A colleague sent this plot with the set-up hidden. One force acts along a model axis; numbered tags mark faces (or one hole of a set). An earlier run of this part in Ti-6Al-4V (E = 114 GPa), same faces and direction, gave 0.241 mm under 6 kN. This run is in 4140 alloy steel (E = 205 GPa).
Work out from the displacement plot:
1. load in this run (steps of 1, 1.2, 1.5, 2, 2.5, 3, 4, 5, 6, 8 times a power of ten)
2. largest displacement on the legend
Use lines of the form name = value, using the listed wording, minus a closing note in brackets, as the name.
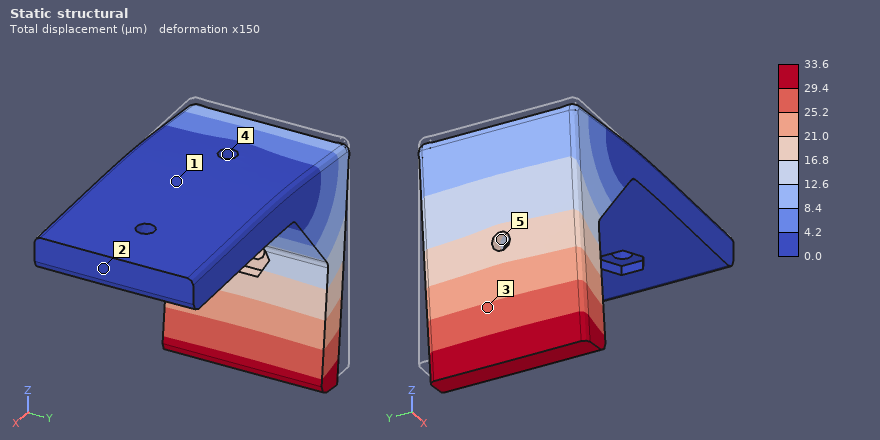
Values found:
load in this run = 1.5 kN
largest displacement on the legend = 33.6 µm
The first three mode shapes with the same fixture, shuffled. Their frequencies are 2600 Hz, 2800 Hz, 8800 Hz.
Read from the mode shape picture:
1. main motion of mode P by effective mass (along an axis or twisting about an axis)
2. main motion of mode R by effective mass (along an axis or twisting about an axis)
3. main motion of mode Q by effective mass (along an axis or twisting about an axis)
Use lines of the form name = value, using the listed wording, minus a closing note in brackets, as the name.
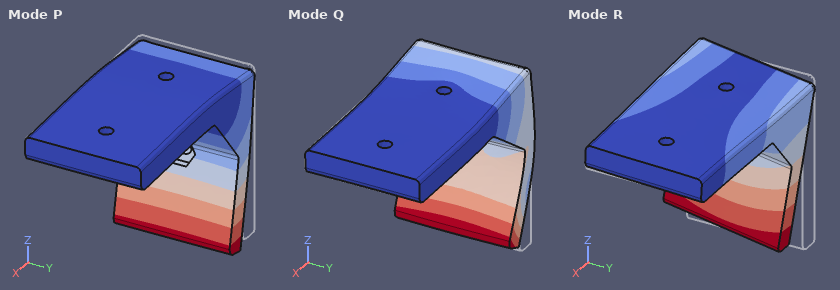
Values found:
main motion of mode P by effective mass = along X
main motion of mode R by effective mass = along Y
main motion of mode Q by effective mass = along Z
